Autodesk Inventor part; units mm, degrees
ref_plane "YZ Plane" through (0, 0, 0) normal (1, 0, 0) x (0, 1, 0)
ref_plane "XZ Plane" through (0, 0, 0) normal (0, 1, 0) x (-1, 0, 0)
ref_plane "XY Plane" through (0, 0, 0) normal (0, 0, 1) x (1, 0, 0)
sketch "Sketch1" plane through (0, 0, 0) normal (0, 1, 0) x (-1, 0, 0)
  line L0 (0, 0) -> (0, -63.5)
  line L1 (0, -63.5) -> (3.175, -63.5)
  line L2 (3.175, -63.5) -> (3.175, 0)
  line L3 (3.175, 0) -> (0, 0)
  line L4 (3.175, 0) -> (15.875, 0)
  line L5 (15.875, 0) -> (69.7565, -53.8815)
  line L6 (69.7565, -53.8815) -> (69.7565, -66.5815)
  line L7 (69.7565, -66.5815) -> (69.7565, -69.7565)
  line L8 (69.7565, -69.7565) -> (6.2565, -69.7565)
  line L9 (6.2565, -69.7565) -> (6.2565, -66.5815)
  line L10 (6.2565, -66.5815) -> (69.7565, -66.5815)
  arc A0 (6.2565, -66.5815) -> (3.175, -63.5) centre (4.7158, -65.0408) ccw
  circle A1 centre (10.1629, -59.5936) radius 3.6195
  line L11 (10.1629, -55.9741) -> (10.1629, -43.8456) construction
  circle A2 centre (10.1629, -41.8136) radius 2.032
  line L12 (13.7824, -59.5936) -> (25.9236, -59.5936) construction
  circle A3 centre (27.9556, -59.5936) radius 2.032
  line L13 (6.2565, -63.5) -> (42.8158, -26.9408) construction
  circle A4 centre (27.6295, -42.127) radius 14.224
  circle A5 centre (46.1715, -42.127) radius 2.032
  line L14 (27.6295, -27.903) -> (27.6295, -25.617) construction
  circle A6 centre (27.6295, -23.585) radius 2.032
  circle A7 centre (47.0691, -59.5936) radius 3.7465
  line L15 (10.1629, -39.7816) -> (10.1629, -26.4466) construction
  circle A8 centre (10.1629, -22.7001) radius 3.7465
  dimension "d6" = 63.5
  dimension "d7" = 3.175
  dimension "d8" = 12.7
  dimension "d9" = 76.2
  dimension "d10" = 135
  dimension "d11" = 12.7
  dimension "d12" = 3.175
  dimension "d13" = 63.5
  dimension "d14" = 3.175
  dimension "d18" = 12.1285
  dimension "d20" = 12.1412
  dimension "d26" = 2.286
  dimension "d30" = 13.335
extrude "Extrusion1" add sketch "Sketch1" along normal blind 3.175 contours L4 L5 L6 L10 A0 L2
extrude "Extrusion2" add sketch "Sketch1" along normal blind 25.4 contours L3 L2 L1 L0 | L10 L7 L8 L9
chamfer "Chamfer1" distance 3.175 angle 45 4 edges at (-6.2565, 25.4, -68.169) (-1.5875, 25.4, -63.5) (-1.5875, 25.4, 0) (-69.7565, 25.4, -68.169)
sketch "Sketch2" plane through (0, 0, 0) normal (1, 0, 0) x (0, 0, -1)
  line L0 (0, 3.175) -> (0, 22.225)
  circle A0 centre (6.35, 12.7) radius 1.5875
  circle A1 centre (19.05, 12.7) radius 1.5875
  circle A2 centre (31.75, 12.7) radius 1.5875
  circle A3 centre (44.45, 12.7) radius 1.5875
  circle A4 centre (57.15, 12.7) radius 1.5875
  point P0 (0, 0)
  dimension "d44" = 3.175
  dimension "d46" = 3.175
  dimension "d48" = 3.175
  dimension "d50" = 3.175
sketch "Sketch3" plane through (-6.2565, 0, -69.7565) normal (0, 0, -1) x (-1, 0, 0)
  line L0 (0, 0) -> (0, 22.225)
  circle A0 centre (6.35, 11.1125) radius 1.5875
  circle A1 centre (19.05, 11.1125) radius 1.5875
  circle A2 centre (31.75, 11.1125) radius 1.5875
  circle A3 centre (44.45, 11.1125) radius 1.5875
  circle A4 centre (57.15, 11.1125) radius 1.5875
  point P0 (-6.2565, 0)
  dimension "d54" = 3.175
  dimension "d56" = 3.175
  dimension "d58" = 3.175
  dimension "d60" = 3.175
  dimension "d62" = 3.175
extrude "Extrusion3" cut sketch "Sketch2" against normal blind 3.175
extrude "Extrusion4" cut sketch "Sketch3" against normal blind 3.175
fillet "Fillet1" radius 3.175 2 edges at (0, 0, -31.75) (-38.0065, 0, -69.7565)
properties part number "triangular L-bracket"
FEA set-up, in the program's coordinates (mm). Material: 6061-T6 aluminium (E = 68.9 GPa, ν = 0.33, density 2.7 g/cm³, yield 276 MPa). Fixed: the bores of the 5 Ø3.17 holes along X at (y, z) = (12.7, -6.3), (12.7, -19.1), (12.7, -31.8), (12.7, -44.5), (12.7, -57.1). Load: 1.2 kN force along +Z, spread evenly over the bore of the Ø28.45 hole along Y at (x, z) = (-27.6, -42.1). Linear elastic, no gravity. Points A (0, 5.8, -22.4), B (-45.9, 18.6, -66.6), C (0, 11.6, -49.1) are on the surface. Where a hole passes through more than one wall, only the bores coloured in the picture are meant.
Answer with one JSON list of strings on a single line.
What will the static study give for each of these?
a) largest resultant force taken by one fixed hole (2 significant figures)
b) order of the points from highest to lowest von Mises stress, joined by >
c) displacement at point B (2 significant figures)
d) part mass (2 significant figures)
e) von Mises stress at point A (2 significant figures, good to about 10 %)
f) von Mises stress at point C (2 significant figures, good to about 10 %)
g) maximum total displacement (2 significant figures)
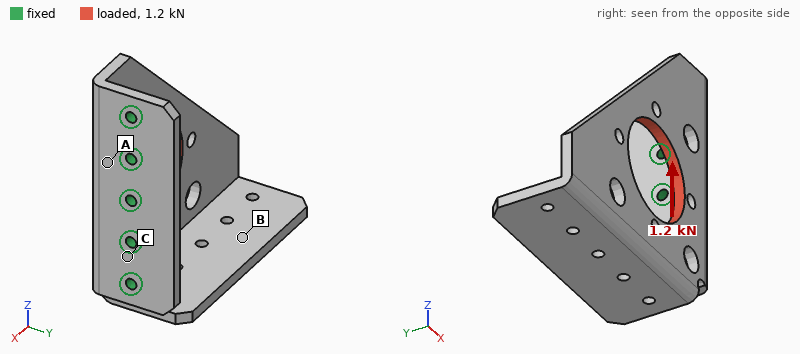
["590 N", "C > A > B", "0.25 mm", "45 g", "31 MPa", "48 MPa", "0.36 mm"]
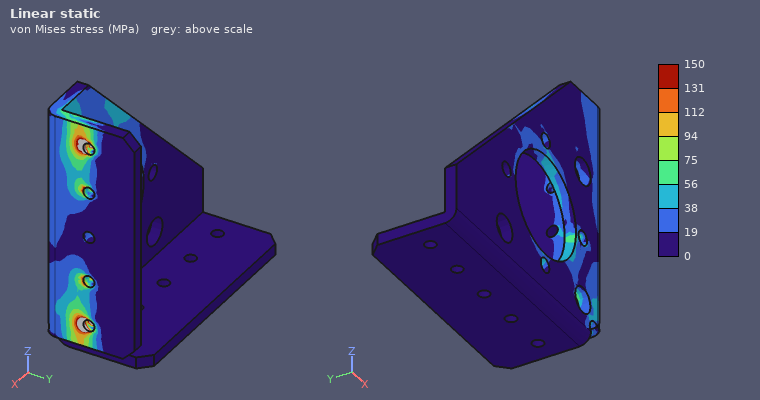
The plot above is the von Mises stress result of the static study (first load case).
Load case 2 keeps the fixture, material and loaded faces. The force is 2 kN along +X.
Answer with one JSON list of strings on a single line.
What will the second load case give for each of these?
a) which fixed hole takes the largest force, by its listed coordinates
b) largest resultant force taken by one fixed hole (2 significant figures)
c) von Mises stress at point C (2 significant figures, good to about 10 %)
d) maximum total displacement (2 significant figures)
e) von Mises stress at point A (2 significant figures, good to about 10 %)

["(12.7, -57.1)", "740 N", "120 MPa", "0.84 mm", "61 MPa"]
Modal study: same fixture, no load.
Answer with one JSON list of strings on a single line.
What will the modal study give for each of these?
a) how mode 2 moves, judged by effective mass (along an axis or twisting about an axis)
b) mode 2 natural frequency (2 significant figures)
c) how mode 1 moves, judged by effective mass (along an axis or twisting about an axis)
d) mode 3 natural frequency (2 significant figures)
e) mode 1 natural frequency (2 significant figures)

["along Z", "1200 Hz", "along Y", "2100 Hz", "370 Hz"]
